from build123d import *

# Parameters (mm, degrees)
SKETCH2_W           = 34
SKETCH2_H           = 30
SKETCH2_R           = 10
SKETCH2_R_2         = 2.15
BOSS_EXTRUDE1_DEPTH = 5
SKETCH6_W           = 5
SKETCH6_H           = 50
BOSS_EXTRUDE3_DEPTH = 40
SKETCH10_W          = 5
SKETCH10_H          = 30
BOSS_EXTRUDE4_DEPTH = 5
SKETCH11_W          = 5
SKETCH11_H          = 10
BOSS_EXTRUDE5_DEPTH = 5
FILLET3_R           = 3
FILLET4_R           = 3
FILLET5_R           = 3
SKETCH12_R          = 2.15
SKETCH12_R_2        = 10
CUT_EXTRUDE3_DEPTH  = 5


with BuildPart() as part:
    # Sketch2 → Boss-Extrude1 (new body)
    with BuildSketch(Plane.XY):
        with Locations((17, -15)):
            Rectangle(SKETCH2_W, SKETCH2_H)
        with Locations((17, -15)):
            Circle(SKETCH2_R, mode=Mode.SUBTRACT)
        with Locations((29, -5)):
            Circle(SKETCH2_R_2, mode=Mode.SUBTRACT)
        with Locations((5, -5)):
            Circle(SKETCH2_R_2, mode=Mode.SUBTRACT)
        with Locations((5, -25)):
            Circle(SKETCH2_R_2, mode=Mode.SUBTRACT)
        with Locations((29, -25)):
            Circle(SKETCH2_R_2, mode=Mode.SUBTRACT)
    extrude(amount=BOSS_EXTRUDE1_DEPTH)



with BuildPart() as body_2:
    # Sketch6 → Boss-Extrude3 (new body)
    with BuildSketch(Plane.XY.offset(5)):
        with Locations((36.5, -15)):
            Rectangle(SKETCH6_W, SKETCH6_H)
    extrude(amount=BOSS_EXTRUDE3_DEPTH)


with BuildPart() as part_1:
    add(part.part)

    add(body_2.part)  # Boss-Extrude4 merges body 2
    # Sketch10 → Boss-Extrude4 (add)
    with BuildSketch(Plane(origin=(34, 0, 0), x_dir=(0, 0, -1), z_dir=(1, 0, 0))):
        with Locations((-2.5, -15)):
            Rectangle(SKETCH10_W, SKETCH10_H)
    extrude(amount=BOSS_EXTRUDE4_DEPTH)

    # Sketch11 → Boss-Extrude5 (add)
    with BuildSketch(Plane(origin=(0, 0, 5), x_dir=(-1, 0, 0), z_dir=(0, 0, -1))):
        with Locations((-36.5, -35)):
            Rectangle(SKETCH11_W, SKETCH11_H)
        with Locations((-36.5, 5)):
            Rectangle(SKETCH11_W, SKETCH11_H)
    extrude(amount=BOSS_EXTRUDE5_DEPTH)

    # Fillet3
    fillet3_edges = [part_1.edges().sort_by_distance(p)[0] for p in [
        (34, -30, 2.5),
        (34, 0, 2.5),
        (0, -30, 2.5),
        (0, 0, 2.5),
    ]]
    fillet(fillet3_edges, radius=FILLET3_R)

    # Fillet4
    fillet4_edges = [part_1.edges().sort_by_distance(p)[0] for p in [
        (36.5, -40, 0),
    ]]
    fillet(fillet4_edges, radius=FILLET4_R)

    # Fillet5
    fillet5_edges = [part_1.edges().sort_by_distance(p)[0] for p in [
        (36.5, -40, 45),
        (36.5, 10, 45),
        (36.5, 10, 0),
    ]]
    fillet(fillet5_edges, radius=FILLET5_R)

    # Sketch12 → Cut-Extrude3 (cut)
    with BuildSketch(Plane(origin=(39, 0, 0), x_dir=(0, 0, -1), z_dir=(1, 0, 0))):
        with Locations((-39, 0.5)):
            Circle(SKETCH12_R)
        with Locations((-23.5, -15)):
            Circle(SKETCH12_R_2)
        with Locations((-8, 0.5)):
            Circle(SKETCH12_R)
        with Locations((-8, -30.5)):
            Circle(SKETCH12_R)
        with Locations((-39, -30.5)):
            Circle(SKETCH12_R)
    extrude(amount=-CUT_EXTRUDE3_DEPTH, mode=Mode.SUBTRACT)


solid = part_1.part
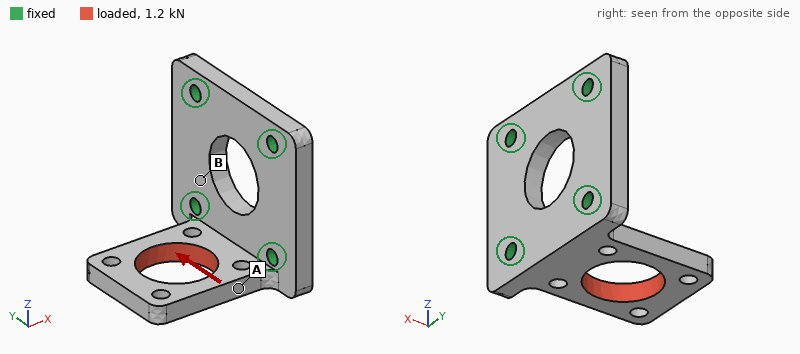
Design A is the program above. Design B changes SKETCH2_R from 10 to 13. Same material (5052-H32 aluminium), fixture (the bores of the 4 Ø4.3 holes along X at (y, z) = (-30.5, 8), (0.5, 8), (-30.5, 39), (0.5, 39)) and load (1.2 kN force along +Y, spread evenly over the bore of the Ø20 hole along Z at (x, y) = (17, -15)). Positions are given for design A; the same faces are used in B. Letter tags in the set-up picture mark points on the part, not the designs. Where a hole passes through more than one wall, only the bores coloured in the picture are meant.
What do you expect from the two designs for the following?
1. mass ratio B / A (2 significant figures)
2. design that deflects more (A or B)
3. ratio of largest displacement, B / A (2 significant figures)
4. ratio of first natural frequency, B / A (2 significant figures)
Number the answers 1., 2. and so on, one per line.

1. 0.91
2. B
3. 4.3
4. 0.87
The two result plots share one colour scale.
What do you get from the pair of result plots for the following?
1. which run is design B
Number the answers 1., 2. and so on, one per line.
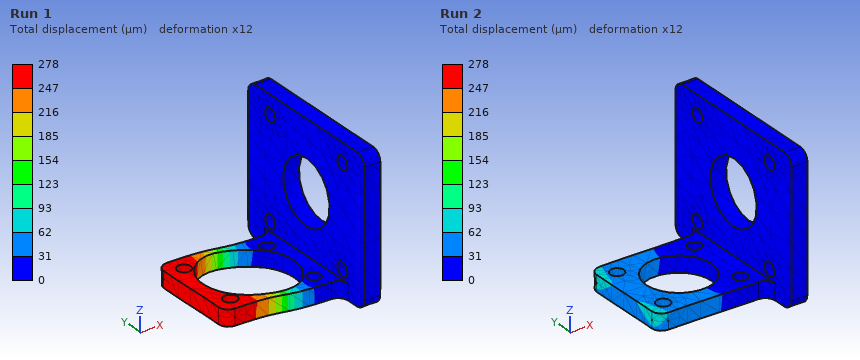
1. Run 1
